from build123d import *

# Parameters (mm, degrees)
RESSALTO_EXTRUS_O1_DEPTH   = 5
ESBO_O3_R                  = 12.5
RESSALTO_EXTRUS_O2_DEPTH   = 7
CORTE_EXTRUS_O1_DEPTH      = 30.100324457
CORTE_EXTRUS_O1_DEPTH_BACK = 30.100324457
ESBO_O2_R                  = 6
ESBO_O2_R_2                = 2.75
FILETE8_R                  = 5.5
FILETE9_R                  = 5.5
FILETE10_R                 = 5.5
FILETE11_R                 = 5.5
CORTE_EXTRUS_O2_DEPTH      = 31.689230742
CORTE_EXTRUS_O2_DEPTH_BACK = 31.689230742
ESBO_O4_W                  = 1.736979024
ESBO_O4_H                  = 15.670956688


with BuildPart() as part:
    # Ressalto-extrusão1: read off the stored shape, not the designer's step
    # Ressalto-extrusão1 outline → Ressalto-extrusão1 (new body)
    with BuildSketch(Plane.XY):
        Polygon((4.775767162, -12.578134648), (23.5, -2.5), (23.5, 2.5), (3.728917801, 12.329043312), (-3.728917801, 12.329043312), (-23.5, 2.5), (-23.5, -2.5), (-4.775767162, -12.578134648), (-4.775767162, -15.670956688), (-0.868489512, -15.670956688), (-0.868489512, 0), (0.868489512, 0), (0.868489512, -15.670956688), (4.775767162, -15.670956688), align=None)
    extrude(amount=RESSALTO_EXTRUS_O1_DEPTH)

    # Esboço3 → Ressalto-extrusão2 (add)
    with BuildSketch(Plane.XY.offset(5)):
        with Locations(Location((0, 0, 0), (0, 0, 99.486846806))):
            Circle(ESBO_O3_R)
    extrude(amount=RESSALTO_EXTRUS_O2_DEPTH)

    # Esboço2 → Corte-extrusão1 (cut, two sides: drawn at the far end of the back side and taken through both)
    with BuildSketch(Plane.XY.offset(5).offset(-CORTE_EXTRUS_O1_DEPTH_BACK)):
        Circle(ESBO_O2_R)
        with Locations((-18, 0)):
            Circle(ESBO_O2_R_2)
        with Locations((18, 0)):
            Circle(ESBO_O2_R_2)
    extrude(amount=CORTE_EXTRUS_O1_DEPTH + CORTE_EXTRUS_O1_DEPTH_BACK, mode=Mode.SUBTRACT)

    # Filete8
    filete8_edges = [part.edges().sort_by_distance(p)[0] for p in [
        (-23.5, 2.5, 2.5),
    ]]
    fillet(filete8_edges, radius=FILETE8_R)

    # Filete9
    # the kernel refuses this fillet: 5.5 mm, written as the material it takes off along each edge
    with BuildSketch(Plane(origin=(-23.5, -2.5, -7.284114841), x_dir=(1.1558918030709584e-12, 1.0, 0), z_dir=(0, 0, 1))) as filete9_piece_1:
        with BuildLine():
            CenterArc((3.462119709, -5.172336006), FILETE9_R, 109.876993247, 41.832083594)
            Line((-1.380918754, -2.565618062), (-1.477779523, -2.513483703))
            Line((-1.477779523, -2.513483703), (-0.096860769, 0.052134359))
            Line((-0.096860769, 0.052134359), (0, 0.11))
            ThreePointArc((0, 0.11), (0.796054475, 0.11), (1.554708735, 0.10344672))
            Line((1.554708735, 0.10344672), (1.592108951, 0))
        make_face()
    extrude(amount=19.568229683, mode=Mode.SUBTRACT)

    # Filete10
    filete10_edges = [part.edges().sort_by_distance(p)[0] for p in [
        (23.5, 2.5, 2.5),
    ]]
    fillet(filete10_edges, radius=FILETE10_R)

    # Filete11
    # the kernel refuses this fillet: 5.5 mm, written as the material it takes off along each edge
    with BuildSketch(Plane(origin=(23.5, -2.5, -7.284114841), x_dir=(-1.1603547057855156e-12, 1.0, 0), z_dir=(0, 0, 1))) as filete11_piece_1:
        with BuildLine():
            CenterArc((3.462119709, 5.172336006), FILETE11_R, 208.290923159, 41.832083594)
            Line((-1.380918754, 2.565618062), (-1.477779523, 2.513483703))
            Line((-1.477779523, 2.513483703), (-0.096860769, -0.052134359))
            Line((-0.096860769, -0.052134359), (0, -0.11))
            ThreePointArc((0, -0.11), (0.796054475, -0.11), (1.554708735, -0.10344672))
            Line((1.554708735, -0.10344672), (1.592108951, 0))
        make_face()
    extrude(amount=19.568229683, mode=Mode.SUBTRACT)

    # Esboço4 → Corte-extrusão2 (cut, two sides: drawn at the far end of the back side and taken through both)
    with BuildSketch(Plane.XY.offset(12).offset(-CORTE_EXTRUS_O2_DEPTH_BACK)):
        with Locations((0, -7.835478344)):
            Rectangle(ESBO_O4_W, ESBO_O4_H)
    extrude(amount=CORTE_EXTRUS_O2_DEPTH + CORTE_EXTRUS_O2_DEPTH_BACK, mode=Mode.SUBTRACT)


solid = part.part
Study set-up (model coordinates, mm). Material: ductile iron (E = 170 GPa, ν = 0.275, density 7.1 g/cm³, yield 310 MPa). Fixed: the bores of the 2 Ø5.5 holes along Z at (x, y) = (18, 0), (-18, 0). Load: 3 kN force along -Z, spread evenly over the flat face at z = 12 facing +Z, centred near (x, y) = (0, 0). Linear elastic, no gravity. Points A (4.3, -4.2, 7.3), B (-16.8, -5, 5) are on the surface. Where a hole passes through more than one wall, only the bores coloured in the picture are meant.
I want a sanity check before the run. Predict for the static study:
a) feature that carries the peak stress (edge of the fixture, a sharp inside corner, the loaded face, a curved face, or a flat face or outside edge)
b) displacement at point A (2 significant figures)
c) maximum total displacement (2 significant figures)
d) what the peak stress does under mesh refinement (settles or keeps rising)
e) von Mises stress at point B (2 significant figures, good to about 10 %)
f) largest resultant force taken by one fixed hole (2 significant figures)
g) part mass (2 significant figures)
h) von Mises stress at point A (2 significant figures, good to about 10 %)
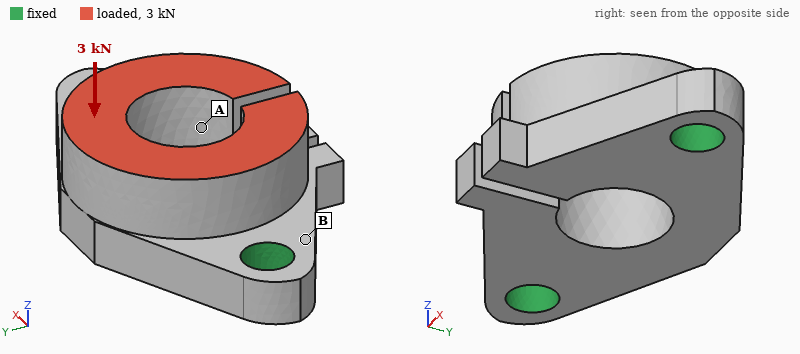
edge of the fixture
14 µm
22 µm
keeps rising
67 MPa
1.6 kN
41 g
26 MPa
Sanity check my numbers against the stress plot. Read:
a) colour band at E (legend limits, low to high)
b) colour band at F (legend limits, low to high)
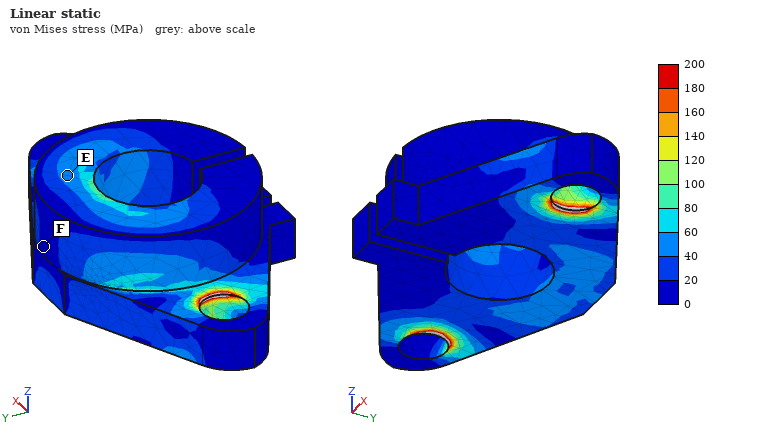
40 to 60 MPa
0 to 20 MPa
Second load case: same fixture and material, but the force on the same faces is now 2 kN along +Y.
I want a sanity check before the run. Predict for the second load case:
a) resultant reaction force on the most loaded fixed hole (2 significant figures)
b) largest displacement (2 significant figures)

1.2 kN
29 µm
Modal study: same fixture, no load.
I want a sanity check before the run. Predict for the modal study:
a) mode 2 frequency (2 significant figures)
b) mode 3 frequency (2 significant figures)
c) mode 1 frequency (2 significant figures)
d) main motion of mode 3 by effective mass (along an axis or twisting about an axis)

12 kHz
13 kHz
10 kHz
along Z
